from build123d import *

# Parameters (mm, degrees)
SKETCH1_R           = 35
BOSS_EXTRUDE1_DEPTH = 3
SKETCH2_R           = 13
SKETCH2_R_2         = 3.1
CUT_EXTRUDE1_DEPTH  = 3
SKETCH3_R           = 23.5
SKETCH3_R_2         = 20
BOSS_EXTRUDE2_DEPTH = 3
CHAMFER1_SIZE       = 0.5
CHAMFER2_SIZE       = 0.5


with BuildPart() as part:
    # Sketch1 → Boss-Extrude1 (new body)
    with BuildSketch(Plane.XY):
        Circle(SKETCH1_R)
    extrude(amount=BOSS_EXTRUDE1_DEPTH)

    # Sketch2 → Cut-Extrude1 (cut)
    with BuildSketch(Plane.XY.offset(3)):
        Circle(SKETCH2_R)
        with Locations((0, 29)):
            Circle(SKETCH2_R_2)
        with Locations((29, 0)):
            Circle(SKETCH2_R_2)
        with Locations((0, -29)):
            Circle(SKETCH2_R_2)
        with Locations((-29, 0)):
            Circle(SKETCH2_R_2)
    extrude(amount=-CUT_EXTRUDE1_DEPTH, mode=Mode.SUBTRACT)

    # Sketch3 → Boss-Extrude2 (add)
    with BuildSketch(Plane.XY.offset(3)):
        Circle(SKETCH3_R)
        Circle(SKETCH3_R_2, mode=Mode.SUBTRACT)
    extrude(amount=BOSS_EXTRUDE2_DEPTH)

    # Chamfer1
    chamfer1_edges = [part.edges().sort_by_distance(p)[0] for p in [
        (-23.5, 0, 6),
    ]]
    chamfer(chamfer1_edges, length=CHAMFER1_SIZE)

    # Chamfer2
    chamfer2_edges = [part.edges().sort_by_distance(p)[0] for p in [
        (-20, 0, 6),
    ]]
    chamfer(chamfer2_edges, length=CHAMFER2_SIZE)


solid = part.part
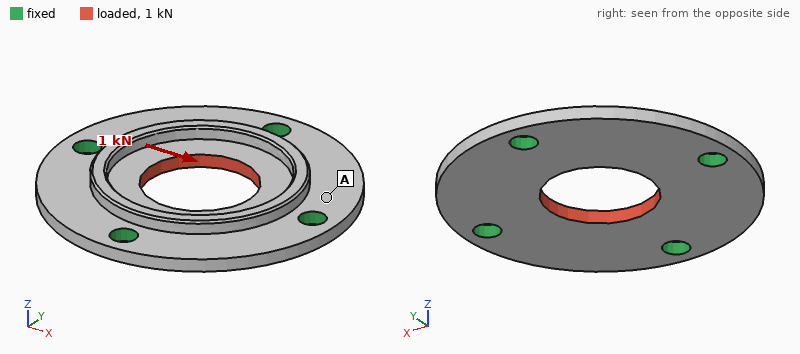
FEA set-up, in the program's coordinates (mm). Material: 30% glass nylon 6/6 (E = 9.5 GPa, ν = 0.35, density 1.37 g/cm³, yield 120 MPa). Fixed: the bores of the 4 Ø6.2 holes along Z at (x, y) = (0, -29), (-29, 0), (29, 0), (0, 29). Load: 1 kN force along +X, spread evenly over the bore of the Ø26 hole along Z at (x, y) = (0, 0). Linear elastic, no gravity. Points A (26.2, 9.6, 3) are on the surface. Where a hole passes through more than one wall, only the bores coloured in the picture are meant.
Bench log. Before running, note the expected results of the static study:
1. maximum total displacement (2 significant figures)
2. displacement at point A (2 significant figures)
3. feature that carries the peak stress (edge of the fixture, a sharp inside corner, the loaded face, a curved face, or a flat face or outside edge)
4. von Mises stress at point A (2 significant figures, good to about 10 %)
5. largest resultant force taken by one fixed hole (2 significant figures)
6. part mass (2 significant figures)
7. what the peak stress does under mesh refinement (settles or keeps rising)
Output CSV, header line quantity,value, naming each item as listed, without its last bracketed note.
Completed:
quantity,value
maximum total displacement,14 µm
displacement at point A,5.8 µm
feature that carries the peak stress,edge of the fixture
von Mises stress at point A,2.2 MPa
largest resultant force taken by one fixed hole,290 N
part mass,15 g
what the peak stress does under mesh refinement,keeps rising
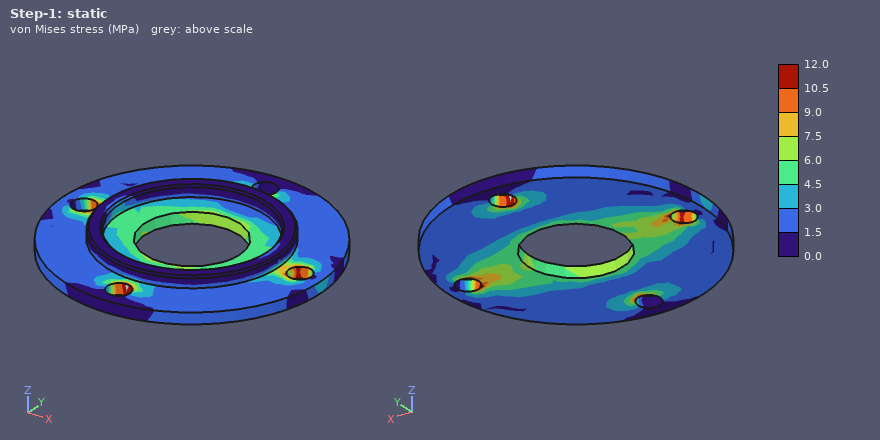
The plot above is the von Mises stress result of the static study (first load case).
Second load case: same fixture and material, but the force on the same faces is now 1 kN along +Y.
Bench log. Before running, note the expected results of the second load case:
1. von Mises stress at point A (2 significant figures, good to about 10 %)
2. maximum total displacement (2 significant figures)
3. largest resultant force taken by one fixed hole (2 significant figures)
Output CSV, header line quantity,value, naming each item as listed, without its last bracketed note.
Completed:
quantity,value
von Mises stress at point A,2.6 MPa
maximum total displacement,14 µm
largest resultant force taken by one fixed hole,290 N
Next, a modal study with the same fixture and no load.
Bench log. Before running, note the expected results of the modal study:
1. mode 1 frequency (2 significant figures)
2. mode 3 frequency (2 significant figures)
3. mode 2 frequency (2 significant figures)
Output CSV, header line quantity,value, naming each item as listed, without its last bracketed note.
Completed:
quantity,value
mode 1 frequency,4800 Hz
mode 3 frequency,5100 Hz
mode 2 frequency,5100 Hz
